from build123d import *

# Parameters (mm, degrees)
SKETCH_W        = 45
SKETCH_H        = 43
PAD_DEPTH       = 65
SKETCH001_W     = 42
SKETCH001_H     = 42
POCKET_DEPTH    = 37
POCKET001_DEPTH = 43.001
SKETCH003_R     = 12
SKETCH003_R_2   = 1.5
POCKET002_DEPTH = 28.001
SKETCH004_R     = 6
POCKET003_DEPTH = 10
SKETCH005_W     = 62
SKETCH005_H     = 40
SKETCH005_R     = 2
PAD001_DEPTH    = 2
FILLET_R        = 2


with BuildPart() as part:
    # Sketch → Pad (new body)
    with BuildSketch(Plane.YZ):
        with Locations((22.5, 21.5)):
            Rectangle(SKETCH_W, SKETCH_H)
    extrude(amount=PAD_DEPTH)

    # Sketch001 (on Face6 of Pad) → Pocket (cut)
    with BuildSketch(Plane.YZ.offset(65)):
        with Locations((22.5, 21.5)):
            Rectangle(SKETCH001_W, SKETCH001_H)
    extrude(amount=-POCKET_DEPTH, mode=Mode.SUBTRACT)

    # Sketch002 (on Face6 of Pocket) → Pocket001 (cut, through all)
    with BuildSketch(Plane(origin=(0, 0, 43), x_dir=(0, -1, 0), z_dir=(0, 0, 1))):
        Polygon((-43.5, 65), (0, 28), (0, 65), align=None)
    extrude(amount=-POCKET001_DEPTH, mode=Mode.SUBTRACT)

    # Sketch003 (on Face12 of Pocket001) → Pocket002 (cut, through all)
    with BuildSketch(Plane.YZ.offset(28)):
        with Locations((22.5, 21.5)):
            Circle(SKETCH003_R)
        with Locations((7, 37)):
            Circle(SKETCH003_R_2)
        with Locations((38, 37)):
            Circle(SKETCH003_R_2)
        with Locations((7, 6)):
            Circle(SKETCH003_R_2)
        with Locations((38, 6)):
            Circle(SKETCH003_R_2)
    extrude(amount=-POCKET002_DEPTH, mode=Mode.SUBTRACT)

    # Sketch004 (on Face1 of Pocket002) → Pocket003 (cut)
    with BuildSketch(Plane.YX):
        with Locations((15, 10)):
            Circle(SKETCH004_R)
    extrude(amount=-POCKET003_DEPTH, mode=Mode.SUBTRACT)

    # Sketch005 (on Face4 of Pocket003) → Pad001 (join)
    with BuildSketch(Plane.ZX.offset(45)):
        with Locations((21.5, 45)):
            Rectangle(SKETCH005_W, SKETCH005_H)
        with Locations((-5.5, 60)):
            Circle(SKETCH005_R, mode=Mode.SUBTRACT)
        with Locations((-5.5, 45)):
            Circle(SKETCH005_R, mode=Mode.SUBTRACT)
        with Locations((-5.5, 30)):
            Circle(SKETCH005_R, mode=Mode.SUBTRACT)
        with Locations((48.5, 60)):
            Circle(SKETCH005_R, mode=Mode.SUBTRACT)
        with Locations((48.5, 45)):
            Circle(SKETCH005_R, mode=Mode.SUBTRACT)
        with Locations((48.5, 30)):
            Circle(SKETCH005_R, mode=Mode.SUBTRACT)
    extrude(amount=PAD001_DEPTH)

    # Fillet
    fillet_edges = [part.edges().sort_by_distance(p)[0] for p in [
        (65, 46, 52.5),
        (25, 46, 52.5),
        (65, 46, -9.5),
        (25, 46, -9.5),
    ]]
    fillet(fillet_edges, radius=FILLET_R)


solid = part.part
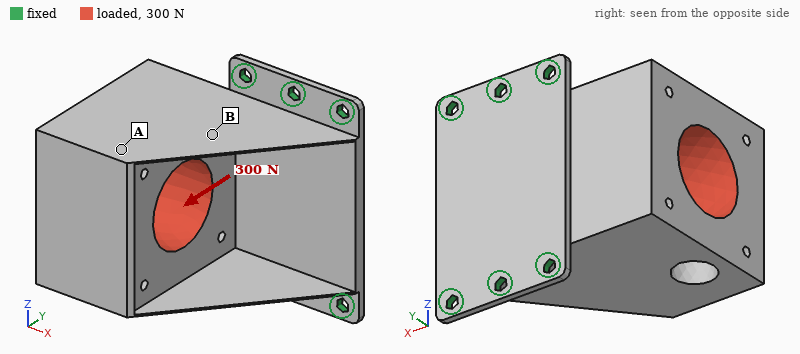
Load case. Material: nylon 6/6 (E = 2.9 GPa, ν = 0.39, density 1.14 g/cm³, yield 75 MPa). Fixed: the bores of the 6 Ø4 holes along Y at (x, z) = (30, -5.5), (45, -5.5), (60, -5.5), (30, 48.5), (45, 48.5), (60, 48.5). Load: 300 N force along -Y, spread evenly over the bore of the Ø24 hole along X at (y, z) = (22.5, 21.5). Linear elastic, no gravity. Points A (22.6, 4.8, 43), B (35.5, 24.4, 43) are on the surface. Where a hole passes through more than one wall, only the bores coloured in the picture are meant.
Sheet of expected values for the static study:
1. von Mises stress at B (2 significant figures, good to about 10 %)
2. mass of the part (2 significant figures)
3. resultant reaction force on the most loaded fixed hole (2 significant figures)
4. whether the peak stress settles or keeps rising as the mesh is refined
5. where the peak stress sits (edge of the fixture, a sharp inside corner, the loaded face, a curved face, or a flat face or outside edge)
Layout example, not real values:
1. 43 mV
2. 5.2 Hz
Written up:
1. 9.4 MPa
2. 54 g
3. 260 N
4. keeps rising
5. edge of the fixture
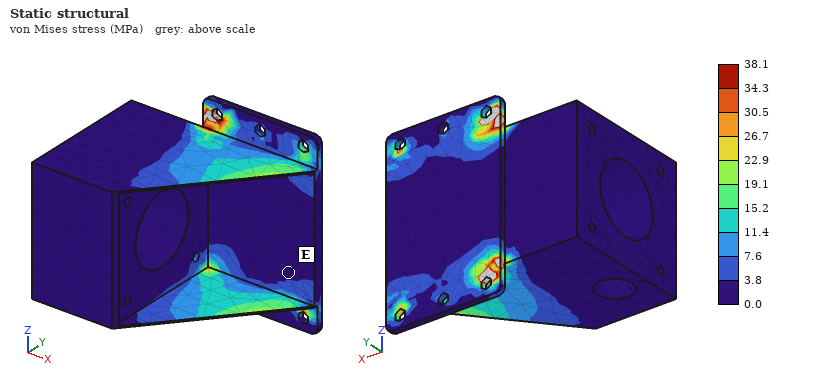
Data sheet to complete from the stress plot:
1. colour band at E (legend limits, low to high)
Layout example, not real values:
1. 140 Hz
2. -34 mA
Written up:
1. 0.0 to 3.8 MPa
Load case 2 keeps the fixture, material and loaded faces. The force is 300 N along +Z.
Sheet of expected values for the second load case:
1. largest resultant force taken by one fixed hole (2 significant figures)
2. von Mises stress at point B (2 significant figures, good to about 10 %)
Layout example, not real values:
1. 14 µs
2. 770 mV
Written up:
1. 160 N
2. 4.9 MPa
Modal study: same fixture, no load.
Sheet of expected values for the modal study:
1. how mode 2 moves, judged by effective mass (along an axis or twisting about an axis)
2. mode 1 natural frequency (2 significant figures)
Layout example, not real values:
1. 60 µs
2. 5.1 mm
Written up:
1. along Z
2. 390 Hz
